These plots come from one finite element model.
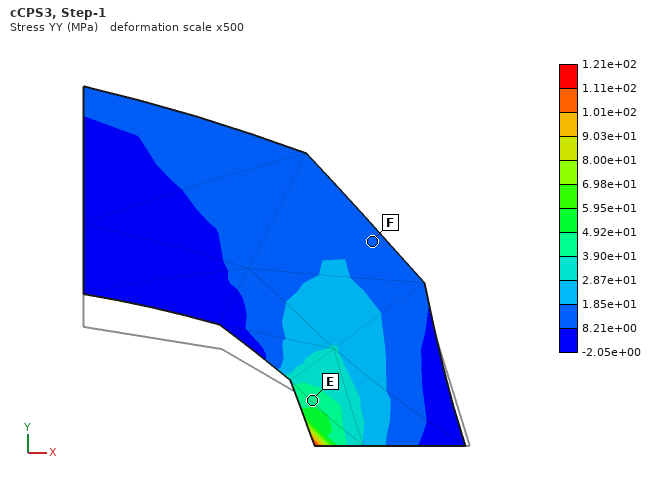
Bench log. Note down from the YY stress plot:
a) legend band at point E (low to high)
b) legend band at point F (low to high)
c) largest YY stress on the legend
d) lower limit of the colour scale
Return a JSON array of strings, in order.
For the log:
["3.90e+01 to 4.92e+01 MPa", "8.21e+00 to 1.85e+01 MPa", "1.21e+02 MPa", "-2.05e+00 MPa"]
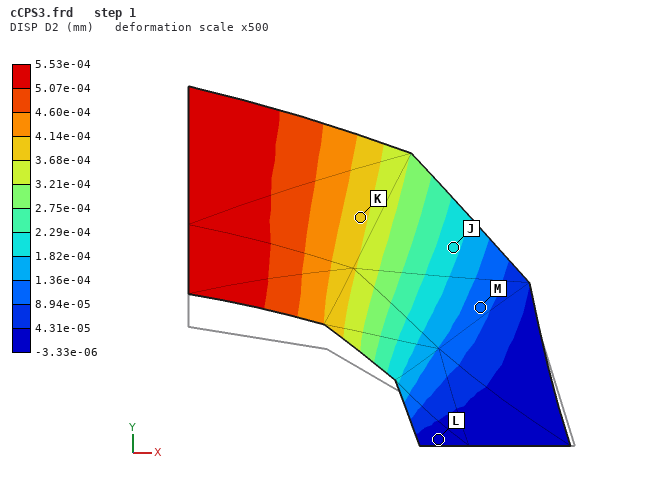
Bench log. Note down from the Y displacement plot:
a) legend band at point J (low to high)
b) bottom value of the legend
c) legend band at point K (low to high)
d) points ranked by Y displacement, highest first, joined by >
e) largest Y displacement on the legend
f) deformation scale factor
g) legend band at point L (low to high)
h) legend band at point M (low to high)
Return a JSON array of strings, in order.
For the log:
["1.82e-04 to 2.29e-04 mm", "-3.33e-06 mm", "3.68e-04 to 4.14e-04 mm", "K > J > M > L", "5.53e-04 mm", "500", "-3.33e-06 to 4.31e-05 mm", "8.94e-05 to 1.36e-04 mm"]
